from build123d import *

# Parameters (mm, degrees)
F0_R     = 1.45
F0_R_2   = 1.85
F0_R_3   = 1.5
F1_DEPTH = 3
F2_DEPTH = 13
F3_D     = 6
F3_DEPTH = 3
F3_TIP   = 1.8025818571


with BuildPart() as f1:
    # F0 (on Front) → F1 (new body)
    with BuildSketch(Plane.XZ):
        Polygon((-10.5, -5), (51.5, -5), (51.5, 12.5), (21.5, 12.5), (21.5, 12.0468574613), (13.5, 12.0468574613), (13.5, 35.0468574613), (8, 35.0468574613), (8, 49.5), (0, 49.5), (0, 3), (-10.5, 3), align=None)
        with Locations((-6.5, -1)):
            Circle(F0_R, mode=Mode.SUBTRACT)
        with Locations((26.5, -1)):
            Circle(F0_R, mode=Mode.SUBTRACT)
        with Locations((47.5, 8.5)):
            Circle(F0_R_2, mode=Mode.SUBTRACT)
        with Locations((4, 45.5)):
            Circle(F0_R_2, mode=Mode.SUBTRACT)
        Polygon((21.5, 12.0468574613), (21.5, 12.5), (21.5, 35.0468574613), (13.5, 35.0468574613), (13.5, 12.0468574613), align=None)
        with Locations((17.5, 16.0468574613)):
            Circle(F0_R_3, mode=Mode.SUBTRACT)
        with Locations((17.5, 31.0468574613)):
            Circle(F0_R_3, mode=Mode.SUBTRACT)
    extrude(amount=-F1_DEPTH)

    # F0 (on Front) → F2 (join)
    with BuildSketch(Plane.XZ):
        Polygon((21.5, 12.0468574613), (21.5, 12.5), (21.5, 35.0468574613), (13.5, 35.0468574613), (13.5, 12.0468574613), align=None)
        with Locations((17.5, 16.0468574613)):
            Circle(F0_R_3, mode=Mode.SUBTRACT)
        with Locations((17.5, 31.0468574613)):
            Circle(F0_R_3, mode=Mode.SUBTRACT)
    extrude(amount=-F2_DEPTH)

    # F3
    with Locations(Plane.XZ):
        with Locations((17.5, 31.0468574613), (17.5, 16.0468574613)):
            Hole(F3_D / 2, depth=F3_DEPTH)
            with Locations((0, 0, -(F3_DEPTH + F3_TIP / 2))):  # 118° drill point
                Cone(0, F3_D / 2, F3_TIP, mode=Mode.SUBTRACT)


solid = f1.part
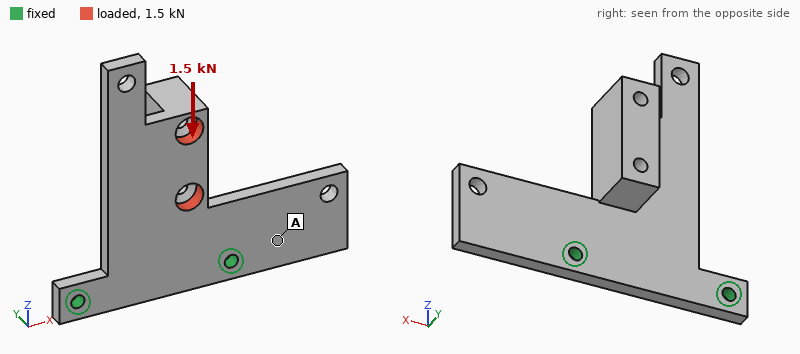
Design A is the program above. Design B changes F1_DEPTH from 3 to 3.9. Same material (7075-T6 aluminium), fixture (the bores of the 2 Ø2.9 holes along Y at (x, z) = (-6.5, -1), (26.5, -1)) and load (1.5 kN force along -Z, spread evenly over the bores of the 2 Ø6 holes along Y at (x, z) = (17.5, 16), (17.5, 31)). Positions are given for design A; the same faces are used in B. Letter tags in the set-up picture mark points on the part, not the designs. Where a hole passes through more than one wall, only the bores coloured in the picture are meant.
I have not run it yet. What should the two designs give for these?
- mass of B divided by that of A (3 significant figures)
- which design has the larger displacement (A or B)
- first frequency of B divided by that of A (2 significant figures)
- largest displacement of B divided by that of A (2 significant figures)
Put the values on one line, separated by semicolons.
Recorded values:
1.20; B; 1.3; 1.9
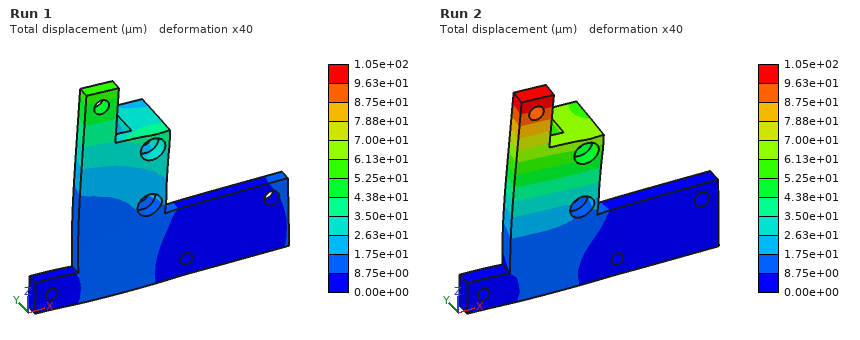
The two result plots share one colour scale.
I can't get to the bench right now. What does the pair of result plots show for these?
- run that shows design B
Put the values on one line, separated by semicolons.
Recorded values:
Run 2
